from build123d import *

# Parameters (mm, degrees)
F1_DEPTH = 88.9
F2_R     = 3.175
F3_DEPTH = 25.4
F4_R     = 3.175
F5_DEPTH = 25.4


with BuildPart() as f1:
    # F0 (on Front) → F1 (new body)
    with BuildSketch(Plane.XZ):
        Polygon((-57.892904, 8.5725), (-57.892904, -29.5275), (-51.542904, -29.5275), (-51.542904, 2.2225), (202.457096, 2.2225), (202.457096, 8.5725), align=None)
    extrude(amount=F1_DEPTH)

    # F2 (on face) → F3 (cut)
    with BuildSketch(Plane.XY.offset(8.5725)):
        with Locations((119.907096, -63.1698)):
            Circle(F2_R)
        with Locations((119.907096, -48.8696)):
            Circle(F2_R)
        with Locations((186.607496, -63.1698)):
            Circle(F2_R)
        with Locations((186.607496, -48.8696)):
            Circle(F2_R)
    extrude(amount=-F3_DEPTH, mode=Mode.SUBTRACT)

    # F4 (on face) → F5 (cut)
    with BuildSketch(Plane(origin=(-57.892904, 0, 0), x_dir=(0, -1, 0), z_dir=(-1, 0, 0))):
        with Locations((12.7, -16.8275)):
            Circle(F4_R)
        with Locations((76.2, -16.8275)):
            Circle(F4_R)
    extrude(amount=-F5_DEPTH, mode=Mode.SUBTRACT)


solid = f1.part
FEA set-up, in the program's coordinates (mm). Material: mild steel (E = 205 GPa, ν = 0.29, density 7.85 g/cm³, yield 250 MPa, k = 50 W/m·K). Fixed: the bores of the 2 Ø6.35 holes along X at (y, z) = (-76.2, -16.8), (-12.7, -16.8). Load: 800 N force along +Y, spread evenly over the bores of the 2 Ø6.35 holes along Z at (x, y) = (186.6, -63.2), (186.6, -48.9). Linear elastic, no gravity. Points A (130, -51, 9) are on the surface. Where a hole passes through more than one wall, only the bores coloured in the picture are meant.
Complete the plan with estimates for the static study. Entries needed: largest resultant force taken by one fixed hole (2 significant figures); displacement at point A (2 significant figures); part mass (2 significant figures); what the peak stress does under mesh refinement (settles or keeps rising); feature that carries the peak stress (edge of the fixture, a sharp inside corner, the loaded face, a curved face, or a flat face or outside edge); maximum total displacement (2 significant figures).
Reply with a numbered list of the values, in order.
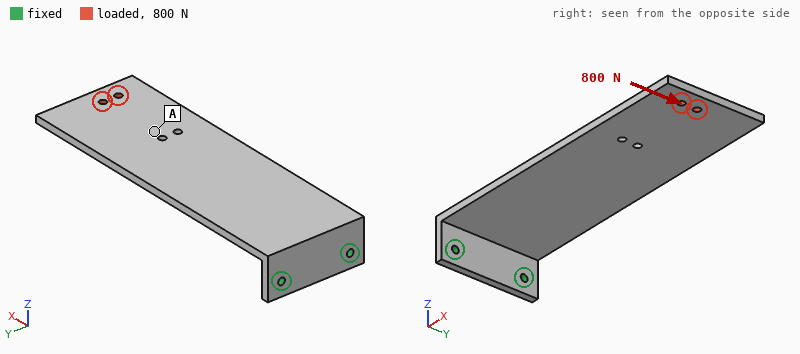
1. 2.9 kN
2. 0.28 mm
3. 1.3 kg
4. keeps rising
5. edge of the fixture
6. 0.43 mm
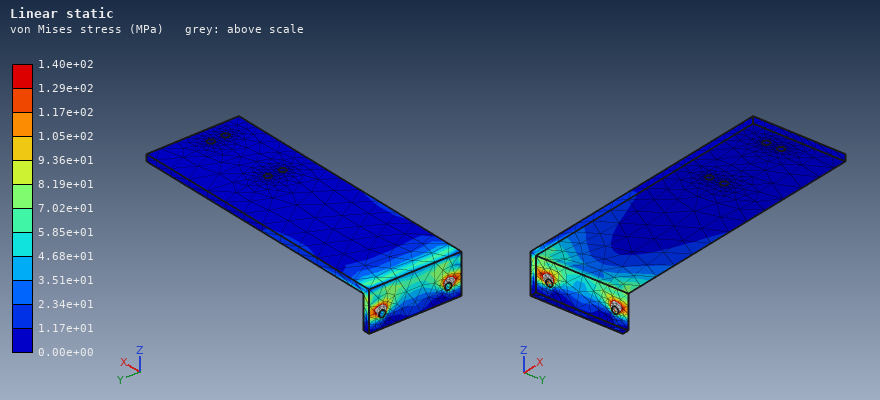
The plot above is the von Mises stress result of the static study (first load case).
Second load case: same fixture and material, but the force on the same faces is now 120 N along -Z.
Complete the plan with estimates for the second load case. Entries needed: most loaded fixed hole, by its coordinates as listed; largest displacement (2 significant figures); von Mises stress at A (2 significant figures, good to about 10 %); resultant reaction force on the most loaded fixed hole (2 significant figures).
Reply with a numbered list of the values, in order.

1. (-76.2, -16.8)
2. 2.0 mm
3. 11 MPa
4. 140 N
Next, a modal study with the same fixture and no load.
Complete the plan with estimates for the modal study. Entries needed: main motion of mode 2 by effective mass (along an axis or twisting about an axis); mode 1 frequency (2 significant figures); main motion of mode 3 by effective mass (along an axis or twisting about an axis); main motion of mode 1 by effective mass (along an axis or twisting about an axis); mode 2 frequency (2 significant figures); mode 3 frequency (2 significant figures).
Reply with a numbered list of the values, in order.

1. along Y
2. 70 Hz
3. along Z
4. along Z
5. 340 Hz
6. 440 Hz
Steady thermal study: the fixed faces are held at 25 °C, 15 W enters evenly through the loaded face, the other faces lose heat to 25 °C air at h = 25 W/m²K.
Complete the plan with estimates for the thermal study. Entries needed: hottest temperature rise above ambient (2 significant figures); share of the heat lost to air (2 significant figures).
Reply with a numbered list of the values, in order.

1. 44 K
2. 95 %
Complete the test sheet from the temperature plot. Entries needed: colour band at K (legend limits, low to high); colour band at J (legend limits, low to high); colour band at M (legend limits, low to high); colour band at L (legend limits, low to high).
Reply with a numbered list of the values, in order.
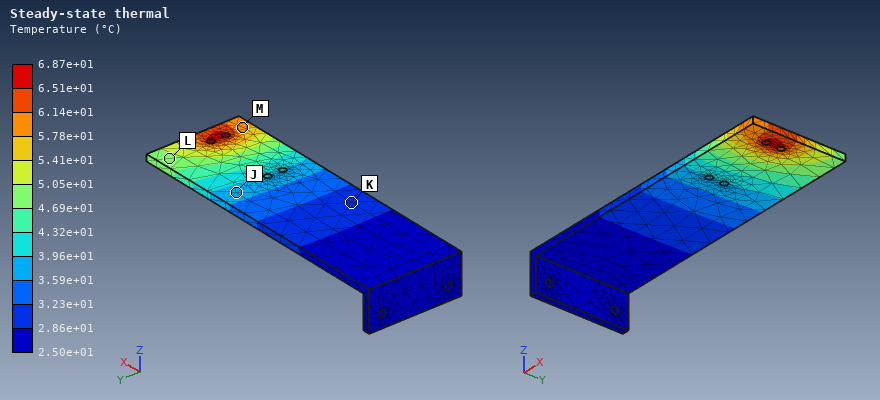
1. 2.86e+01 to 3.23e+01 °C
2. 3.59e+01 to 3.96e+01 °C
3. 5.78e+01 to 6.14e+01 °C
4. 4.69e+01 to 5.05e+01 °C
